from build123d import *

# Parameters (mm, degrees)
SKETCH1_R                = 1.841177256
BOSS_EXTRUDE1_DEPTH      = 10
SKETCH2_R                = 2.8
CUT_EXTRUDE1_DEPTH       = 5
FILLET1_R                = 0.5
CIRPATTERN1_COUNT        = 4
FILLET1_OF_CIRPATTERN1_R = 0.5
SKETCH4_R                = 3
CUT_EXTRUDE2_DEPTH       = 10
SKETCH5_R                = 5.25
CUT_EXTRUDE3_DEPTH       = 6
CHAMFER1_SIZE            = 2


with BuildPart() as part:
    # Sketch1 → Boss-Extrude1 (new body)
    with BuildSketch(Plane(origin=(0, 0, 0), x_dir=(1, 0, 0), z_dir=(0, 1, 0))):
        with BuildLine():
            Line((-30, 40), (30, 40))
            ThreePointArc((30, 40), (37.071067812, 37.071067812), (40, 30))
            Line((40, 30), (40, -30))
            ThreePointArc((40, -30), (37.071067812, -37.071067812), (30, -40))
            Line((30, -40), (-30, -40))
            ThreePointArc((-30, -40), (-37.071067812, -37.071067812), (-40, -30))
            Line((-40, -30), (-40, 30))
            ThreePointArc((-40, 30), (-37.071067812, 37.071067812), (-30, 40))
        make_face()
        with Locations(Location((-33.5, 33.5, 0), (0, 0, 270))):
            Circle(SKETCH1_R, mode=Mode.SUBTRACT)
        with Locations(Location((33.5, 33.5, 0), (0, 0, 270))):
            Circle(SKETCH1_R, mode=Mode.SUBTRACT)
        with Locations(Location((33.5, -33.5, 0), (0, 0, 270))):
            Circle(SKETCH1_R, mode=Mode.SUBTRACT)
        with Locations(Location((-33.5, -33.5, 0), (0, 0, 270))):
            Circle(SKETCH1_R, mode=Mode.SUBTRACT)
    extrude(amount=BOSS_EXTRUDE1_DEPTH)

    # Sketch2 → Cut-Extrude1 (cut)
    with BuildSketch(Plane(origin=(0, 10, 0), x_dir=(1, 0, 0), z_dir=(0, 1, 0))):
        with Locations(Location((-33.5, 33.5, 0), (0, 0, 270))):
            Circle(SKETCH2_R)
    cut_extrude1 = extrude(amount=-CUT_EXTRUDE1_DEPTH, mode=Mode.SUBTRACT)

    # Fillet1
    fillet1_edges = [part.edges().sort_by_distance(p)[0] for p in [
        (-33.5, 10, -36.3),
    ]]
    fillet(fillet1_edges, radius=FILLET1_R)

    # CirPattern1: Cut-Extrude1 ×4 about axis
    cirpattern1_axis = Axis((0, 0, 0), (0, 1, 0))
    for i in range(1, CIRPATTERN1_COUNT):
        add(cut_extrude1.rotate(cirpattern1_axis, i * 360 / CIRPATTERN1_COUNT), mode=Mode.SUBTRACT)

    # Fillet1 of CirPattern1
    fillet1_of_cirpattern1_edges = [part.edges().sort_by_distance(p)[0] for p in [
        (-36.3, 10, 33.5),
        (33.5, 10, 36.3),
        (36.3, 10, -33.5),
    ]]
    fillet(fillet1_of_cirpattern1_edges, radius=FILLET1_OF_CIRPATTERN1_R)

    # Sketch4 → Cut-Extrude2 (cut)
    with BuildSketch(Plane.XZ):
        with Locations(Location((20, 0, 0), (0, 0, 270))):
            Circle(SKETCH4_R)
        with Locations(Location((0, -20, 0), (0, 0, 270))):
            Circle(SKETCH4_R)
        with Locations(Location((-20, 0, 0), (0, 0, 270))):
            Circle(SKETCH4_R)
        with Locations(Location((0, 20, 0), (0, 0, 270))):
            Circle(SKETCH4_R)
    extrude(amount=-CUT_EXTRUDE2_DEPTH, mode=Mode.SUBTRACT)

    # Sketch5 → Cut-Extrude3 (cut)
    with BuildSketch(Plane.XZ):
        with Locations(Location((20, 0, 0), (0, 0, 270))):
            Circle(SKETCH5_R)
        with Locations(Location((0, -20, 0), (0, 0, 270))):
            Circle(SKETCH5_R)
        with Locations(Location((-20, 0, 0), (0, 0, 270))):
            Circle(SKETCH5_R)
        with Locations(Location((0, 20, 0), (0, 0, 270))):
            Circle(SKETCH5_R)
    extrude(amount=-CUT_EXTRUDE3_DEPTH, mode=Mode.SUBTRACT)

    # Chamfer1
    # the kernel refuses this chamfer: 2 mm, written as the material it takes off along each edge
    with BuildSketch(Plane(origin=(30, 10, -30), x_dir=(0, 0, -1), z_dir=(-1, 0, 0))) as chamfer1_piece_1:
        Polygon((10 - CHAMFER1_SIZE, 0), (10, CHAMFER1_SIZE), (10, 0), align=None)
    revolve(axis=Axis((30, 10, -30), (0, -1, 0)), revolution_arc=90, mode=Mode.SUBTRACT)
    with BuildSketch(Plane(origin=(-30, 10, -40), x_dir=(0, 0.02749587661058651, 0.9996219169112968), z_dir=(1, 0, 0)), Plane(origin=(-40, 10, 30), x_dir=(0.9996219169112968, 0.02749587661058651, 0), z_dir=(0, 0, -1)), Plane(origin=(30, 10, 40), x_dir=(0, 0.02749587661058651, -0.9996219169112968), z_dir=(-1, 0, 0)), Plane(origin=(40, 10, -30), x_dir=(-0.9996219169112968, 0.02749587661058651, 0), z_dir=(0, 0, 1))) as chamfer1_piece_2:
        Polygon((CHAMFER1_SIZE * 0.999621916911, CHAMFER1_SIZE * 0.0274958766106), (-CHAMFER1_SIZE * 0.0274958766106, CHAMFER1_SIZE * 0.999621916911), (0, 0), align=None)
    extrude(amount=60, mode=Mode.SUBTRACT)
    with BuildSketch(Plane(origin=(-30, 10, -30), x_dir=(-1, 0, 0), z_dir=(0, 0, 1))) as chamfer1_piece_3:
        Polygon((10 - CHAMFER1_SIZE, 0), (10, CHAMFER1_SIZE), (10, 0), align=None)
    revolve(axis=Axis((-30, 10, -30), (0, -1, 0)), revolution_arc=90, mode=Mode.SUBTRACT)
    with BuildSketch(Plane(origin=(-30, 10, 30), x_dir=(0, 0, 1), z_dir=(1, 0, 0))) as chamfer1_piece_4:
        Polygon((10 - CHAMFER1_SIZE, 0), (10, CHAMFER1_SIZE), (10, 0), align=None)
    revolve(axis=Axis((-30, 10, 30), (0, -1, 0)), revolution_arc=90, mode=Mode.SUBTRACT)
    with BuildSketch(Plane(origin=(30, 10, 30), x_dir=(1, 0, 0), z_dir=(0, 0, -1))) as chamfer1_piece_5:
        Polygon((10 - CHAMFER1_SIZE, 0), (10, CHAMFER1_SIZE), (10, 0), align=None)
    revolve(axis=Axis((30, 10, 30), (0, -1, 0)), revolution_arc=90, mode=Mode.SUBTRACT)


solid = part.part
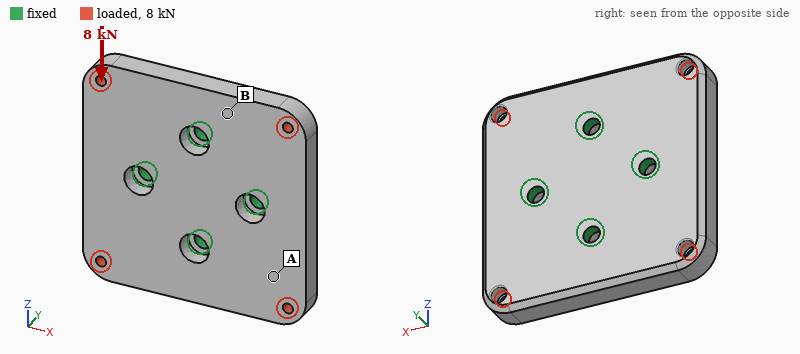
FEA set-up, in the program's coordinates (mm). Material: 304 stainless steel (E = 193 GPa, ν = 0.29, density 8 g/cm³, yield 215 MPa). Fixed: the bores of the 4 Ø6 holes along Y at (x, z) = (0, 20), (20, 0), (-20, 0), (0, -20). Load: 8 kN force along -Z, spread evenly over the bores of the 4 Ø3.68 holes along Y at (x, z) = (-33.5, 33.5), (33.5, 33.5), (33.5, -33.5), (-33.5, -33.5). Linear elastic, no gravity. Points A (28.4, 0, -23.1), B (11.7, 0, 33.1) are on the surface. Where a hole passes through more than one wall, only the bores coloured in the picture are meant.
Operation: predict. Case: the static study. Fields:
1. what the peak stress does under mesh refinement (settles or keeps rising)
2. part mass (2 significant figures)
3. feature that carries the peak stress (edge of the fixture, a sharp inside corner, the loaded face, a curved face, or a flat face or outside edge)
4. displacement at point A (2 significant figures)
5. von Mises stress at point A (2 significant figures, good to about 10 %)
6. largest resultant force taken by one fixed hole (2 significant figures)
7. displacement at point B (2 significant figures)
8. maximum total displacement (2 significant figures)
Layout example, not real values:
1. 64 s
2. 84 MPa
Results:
1. keeps rising
2. 470 g
3. edge of the fixture
4. 4.9 µm
5. 21 MPa
6. 2.8 kN
7. 4.0 µm
8. 11 µm
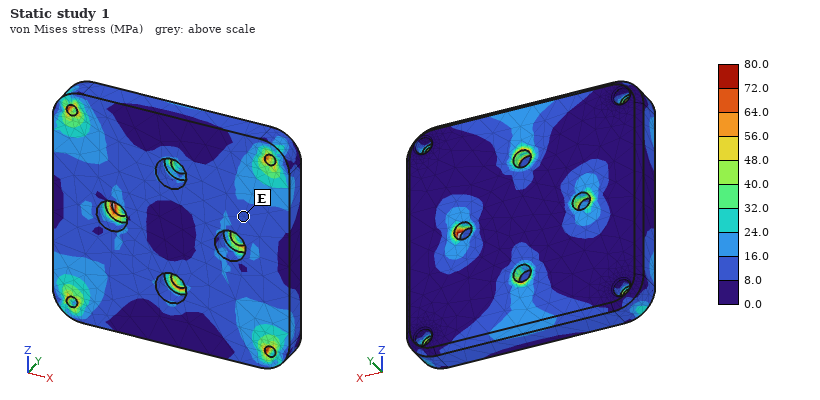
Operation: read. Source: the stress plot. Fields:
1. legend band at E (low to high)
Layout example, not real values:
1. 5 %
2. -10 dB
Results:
1. 8.0 to 16.0 MPa
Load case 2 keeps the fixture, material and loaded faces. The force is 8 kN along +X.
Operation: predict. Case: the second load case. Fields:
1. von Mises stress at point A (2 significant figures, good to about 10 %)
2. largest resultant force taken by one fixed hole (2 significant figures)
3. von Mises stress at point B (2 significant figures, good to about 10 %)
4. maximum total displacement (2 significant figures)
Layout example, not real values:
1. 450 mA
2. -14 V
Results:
1. 17 MPa
2. 2.8 kN
3. 12 MPa
4. 11 µm
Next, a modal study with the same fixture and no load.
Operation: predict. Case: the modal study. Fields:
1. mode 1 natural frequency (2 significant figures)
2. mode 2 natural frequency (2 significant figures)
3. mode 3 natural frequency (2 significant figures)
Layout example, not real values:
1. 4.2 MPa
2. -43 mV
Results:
1. 5800 Hz
2. 6100 Hz
3. 6100 Hz
